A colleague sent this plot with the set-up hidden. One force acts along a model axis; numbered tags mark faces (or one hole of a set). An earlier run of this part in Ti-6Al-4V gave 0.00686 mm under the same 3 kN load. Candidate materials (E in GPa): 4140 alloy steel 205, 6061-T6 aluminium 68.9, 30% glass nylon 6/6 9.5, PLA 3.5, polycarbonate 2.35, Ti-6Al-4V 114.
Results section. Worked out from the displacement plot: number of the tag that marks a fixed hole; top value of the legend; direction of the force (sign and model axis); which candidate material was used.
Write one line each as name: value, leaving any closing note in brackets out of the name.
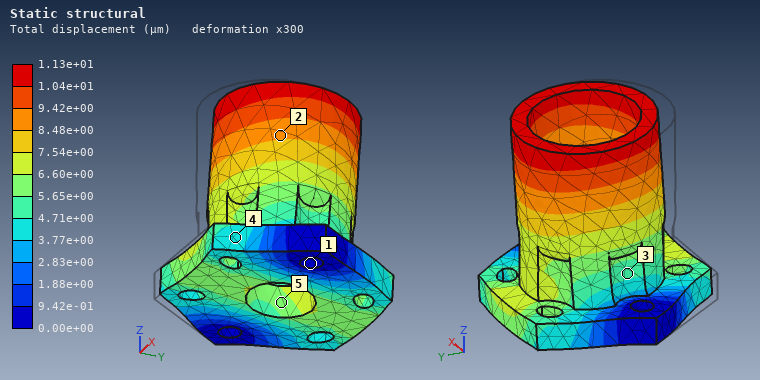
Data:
number of the tag that marks a fixed hole: 1
top value of the legend: 1.13e+01 µm
direction of the force: +Y
which candidate material was used: 6061-T6 aluminium
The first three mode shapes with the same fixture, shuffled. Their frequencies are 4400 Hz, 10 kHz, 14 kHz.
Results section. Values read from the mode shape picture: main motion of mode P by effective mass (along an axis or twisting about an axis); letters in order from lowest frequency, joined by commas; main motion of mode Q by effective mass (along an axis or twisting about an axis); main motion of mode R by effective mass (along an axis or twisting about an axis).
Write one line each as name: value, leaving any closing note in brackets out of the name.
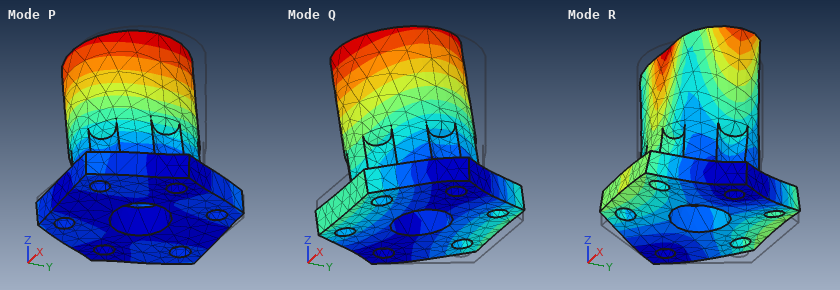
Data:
main motion of mode P by effective mass: along X
letters in order from lowest frequency, joined by commas: Q, P, R
main motion of mode Q by effective mass: along Y
main motion of mode R by effective mass: along Z
